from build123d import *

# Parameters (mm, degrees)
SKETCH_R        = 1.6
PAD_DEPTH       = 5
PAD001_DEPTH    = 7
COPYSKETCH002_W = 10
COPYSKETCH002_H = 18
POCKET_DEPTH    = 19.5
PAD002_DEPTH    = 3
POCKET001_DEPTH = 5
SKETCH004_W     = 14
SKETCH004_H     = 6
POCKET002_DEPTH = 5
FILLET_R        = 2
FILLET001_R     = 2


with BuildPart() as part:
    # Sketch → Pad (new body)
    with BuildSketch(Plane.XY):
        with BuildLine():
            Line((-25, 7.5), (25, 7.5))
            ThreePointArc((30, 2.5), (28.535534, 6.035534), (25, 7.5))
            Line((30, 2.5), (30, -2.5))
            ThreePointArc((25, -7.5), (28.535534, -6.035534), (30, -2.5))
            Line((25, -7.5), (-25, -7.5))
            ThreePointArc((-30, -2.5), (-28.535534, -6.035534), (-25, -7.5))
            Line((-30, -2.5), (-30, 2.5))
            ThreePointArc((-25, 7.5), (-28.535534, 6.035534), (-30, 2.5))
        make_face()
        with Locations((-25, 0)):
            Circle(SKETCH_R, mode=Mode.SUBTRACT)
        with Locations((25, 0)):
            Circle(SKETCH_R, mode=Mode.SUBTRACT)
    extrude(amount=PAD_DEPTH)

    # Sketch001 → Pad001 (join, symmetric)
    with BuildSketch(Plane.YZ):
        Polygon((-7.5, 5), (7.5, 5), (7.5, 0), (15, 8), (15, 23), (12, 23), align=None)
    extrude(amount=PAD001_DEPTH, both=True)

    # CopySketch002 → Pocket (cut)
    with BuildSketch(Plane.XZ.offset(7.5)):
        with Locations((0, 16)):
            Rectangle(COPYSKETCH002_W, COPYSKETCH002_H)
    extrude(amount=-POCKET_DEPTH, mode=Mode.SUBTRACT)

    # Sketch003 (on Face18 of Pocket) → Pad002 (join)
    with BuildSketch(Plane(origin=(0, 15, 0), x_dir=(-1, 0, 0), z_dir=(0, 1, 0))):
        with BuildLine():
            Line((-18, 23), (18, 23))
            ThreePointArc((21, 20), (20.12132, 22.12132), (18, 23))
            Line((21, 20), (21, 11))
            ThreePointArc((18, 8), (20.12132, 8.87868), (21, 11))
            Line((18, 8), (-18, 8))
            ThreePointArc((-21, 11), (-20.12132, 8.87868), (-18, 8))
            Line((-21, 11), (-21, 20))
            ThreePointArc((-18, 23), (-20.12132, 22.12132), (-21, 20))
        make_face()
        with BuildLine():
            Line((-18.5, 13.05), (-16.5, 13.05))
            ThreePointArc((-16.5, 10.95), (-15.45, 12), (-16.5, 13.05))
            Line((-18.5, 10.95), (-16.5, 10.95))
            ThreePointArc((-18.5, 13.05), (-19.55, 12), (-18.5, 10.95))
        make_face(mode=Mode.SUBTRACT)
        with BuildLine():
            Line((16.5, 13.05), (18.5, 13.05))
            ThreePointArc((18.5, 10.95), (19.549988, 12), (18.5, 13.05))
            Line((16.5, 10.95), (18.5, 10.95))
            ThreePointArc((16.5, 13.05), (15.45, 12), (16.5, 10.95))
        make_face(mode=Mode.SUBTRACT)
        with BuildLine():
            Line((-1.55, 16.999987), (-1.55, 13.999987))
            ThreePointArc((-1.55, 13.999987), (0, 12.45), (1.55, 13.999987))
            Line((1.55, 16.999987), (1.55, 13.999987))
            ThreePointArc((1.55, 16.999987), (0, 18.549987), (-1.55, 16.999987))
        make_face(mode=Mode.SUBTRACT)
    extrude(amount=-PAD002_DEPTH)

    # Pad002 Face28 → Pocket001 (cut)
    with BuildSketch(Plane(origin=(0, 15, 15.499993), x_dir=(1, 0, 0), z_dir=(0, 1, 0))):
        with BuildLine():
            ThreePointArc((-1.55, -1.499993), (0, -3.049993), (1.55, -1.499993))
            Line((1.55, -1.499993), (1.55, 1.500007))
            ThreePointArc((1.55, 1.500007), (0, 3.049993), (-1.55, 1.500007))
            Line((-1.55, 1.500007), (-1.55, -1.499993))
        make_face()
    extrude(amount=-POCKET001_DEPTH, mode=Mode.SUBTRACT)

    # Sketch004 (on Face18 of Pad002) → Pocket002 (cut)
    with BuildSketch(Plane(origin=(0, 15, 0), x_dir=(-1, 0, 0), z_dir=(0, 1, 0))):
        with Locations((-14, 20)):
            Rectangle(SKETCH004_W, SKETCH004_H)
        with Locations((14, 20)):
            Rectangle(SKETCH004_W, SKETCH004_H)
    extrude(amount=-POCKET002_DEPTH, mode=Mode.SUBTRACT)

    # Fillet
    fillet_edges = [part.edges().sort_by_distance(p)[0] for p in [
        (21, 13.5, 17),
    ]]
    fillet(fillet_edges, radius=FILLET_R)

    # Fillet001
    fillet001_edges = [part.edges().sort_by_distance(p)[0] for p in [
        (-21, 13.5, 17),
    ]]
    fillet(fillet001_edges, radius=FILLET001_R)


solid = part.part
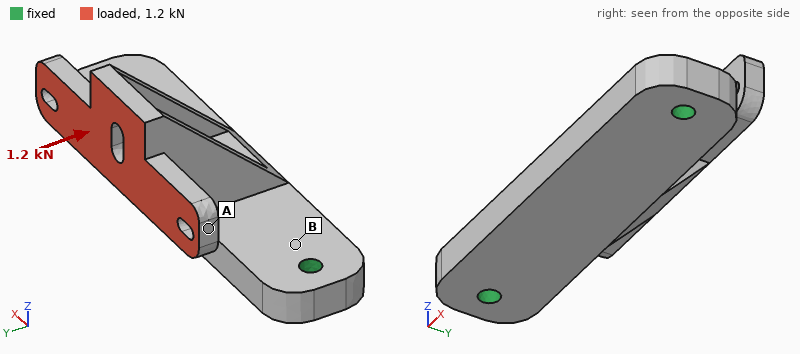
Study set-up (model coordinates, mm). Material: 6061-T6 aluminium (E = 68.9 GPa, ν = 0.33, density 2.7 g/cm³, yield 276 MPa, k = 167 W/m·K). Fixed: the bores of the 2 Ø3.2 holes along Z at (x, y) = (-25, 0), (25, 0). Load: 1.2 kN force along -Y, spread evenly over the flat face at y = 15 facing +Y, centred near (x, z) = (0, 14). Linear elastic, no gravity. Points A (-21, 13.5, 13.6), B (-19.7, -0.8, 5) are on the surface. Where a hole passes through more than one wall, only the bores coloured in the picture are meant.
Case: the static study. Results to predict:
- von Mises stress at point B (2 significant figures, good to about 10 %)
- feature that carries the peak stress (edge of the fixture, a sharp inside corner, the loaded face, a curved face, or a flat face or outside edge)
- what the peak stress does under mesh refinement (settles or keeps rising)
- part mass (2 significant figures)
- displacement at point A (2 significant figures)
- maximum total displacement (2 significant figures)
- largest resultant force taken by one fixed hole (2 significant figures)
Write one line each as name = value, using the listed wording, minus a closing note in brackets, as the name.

von Mises stress at point B = 120 MPa
feature that carries the peak stress = edge of the fixture
what the peak stress does under mesh refinement = keeps rising
part mass = 19 g
displacement at point A = 0.31 mm
maximum total displacement = 0.34 mm
largest resultant force taken by one fixed hole = 600 N
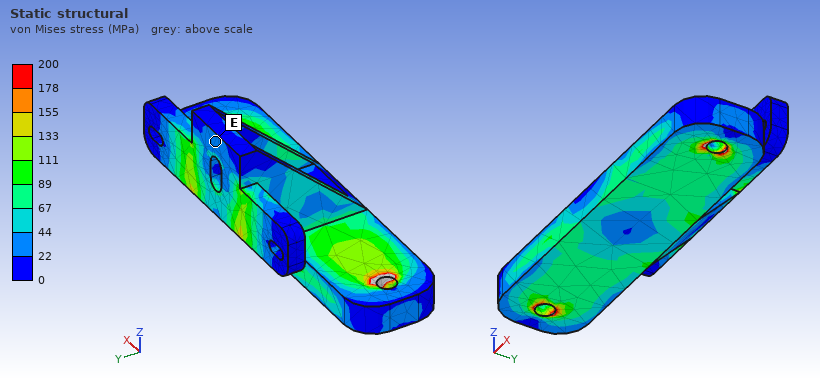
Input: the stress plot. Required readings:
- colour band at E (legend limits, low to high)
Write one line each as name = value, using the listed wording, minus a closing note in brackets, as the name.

colour band at E = 22 to 44 MPa
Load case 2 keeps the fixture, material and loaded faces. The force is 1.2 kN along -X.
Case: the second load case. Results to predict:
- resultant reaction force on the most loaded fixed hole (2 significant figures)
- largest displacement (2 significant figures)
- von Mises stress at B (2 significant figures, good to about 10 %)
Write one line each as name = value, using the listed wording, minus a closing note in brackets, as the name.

resultant reaction force on the most loaded fixed hole = 820 N
largest displacement = 0.15 mm
von Mises stress at B = 11 MPa
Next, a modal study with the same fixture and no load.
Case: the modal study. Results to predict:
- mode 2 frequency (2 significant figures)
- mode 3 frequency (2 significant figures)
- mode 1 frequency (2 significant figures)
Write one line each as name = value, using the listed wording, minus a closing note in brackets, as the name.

mode 2 frequency = 6600 Hz
mode 3 frequency = 7700 Hz
mode 1 frequency = 4200 Hz
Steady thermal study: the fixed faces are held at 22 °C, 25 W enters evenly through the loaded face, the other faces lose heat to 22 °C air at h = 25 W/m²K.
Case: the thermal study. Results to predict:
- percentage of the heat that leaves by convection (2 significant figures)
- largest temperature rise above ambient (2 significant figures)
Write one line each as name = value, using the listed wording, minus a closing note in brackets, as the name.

percentage of the heat that leaves by convection = 8.5 %
largest temperature rise above ambient = 51 K
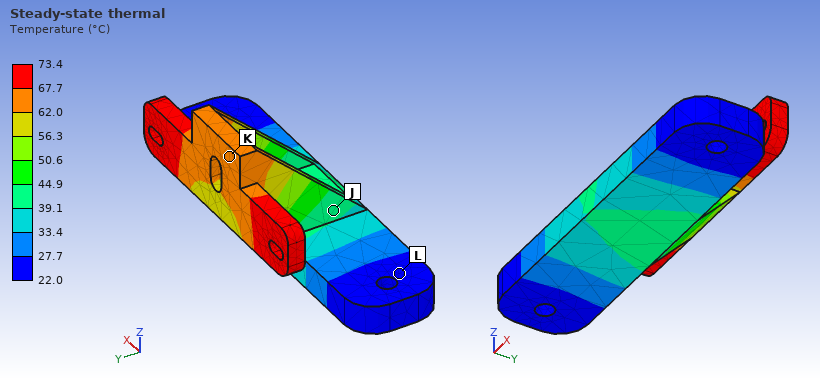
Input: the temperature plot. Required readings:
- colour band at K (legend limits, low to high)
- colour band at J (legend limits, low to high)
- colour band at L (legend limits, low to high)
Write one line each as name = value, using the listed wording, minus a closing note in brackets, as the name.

colour band at K = 62.0 to 67.7 °C
colour band at J = 39.1 to 44.9 °C
colour band at L = 22.0 to 27.7 °C
